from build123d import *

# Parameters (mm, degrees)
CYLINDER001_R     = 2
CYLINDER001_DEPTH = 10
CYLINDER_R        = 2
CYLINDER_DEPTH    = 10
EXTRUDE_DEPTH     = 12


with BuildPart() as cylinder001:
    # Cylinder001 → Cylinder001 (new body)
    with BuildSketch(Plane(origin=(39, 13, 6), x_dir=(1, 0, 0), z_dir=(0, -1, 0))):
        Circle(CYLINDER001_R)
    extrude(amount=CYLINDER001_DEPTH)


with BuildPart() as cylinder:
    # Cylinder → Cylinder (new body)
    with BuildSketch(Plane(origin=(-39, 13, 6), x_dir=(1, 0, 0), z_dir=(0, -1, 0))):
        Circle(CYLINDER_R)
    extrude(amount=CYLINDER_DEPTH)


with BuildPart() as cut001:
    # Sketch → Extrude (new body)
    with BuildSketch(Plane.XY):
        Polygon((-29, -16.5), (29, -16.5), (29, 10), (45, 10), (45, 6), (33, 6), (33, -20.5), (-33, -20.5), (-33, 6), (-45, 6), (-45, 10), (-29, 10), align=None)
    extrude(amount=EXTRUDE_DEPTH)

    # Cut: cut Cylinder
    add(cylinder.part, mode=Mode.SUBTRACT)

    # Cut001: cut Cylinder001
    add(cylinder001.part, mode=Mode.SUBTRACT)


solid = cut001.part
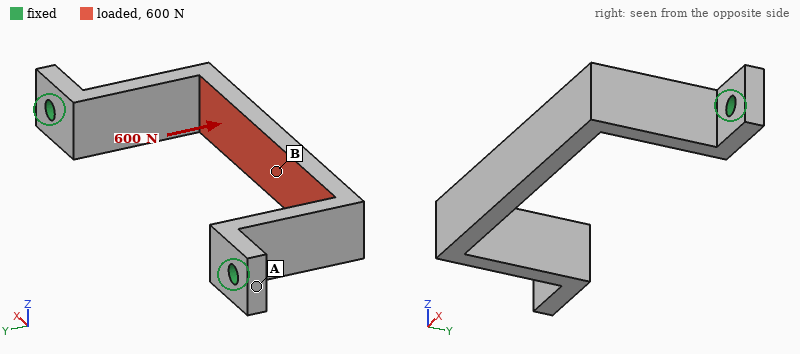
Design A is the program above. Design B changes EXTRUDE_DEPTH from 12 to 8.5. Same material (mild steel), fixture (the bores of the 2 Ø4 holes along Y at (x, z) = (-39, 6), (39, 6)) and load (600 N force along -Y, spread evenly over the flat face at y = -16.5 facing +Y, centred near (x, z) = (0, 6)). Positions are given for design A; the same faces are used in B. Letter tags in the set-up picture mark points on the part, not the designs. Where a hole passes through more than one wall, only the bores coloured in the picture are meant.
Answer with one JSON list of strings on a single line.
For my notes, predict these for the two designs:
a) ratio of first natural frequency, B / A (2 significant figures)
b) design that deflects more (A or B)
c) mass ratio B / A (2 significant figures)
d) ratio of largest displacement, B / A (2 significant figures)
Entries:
["0.87", "B", "0.70", "1.4"]
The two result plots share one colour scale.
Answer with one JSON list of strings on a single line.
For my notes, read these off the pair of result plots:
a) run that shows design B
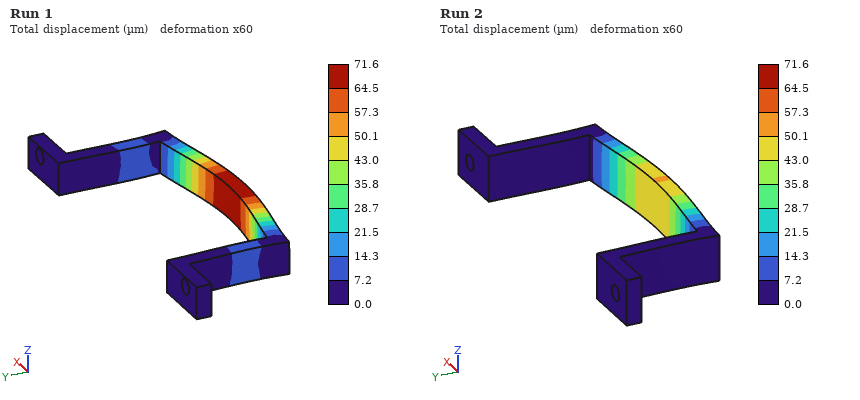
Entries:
["Run 1"]
